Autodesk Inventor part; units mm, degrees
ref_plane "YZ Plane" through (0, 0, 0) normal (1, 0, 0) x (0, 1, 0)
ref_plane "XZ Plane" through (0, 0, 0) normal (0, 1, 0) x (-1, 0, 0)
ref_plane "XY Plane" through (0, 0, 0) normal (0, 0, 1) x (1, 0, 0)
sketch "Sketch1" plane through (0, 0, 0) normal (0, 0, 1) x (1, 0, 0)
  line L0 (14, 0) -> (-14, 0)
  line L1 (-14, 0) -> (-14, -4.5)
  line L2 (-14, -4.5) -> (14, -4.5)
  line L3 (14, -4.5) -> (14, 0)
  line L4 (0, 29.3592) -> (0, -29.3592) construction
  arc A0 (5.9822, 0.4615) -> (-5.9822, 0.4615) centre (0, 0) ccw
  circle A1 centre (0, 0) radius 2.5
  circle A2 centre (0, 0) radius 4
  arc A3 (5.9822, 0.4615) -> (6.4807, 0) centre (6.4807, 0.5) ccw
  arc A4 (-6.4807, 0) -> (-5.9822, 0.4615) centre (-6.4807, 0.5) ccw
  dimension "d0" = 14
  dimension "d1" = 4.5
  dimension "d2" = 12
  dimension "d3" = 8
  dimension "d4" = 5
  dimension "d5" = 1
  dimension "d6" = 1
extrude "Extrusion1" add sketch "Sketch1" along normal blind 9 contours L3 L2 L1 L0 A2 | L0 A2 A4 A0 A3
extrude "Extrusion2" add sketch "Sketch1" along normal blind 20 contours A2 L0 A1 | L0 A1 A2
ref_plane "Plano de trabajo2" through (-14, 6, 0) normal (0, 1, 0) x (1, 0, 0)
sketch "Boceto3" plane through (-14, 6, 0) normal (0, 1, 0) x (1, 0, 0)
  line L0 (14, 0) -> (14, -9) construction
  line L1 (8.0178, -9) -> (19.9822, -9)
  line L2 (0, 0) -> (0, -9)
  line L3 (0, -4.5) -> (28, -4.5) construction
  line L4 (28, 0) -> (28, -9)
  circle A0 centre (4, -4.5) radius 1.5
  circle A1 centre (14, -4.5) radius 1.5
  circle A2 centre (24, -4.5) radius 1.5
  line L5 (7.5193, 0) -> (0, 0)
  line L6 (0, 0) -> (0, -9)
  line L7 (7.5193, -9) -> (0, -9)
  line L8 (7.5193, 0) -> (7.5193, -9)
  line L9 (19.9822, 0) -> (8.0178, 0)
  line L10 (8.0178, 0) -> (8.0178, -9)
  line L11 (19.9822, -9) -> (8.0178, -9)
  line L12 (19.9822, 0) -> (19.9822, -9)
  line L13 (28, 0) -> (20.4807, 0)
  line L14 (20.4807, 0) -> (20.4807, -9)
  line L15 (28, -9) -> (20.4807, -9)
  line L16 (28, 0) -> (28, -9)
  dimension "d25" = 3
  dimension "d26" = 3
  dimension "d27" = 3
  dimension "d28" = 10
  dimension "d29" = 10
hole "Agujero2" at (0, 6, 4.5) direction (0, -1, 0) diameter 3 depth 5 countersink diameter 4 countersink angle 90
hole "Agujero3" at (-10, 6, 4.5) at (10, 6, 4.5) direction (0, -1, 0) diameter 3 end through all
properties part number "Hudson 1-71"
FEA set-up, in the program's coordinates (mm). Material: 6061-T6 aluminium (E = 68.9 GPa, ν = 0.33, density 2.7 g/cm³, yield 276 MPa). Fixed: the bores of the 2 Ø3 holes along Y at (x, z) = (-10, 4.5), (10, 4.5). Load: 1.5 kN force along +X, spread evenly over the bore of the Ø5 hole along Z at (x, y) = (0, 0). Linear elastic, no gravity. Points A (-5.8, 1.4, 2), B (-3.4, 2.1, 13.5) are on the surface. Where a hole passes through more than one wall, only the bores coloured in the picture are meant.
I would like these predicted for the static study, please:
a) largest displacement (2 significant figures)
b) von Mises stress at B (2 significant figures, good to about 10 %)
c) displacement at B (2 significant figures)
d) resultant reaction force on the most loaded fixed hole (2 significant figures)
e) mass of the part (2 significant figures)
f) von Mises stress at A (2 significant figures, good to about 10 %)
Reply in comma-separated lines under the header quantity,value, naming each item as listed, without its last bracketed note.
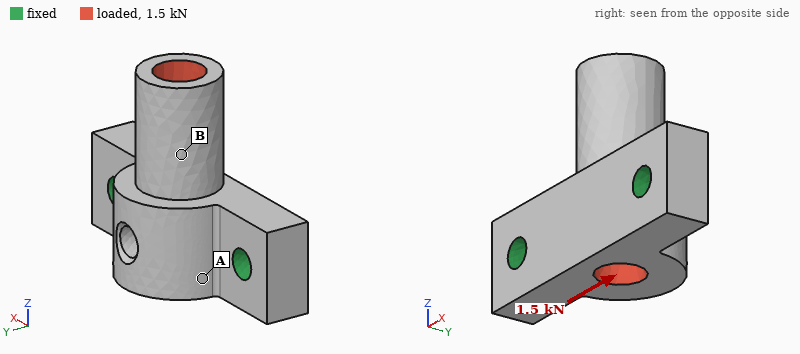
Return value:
quantity,value
largest displacement,42 µm
von Mises stress at B,40 MPa
displacement at B,23 µm
resultant reaction force on the most loaded fixed hole,910 N
mass of the part,4.6 g
von Mises stress at A,19 MPa
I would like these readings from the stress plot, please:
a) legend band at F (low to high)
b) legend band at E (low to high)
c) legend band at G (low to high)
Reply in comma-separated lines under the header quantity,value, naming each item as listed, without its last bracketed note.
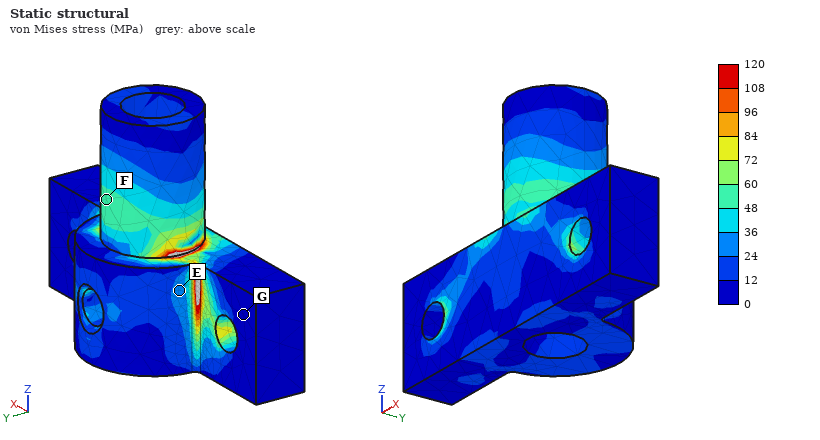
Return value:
quantity,value
legend band at F,48 to 60 MPa
legend band at E,24 to 36 MPa
legend band at G,0 to 12 MPa
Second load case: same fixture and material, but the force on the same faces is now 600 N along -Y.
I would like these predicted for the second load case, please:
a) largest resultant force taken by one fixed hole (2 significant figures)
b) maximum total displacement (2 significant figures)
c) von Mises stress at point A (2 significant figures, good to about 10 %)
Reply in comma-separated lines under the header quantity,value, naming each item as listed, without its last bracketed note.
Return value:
quantity,value
largest resultant force taken by one fixed hole,310 N
maximum total displacement,44 µm
von Mises stress at point A,18 MPa
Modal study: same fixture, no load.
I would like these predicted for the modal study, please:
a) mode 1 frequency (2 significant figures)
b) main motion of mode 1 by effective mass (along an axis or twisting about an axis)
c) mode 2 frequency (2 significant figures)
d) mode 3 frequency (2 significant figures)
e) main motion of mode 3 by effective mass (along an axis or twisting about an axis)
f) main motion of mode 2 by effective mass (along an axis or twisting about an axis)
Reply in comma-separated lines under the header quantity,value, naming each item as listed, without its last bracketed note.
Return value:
quantity,value
mode 1 frequency,16 kHz
main motion of mode 1 by effective mass,along Y
mode 2 frequency,28 kHz
mode 3 frequency,36 kHz
main motion of mode 3 by effective mass,along Z
main motion of mode 2 by effective mass,along X
